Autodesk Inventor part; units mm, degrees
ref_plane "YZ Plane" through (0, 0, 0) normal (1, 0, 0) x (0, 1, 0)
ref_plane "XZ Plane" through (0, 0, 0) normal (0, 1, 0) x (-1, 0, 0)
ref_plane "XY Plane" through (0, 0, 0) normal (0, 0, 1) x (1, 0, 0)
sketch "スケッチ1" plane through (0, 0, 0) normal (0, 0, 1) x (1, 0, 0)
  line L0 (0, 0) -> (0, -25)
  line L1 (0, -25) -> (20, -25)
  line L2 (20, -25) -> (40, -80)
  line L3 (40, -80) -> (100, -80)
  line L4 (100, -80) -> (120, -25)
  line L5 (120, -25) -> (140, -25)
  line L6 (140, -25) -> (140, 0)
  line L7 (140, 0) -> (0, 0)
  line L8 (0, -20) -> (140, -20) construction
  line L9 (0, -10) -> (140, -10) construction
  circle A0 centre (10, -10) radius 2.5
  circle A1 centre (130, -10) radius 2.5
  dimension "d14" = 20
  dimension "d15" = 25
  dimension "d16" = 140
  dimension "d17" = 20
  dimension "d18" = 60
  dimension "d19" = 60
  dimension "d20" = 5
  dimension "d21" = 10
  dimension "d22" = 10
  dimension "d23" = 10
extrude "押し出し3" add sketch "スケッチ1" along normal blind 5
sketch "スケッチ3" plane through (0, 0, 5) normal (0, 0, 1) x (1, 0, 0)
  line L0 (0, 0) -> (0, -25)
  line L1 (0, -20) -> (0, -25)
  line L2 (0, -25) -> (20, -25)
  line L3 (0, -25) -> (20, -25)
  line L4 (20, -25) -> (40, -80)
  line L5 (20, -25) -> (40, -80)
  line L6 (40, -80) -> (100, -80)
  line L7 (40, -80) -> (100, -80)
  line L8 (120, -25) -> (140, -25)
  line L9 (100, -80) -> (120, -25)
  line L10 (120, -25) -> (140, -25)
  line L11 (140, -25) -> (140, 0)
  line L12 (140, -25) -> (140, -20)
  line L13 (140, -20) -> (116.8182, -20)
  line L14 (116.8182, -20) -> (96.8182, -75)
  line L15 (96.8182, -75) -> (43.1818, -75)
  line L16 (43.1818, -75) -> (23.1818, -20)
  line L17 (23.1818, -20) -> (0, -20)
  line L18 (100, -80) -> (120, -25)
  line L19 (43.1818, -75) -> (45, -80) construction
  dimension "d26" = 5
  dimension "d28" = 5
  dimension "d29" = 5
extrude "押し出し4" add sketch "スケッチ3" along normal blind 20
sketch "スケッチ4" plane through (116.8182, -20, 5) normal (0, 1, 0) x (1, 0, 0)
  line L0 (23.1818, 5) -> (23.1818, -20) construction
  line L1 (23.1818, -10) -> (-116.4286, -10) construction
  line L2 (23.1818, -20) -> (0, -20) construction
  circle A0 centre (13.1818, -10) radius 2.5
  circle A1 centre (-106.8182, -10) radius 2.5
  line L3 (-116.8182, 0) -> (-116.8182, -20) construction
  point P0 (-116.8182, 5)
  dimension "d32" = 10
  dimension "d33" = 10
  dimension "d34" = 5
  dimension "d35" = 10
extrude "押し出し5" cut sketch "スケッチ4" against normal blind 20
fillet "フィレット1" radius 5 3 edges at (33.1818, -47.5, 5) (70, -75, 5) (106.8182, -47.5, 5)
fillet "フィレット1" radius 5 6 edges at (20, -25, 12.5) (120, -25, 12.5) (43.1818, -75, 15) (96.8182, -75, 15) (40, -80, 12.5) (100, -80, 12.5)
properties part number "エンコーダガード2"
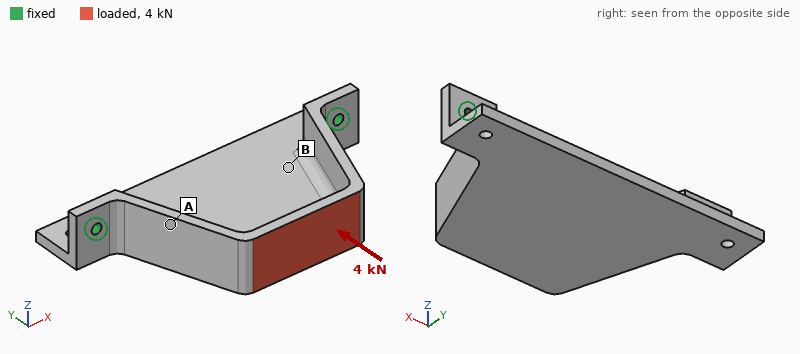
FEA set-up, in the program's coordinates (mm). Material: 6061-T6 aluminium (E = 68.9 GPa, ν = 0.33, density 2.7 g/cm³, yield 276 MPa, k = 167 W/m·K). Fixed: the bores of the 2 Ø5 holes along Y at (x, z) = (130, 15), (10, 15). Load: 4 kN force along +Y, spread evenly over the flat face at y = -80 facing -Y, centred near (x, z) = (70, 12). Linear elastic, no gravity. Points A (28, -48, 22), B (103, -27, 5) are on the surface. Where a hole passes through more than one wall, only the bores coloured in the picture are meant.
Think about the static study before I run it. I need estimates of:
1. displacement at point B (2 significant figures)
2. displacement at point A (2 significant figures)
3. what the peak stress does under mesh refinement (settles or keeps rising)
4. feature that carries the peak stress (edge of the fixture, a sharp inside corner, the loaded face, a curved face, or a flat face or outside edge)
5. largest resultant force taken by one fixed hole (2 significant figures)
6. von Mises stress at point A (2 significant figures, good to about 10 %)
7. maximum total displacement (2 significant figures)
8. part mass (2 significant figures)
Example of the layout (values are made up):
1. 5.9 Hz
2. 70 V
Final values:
1. 0.033 mm
2. 0.039 mm
3. keeps rising
4. edge of the fixture
5. 2.1 kN
6. 27 MPa
7. 0.14 mm
8. 160 g
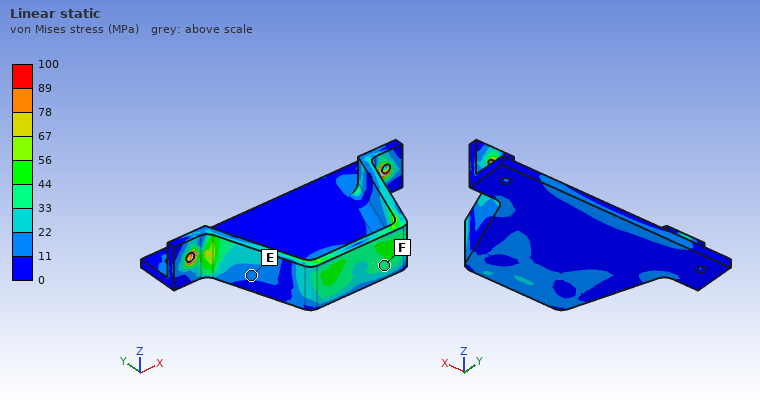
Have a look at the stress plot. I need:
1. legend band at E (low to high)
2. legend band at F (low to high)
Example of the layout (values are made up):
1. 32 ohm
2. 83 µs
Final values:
1. 11 to 22 MPa
2. 33 to 44 MPa
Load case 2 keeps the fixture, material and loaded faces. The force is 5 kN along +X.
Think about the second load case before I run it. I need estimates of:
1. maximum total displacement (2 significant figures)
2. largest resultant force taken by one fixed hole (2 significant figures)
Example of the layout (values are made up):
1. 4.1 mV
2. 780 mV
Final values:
1. 0.45 mm
2. 3.5 kN
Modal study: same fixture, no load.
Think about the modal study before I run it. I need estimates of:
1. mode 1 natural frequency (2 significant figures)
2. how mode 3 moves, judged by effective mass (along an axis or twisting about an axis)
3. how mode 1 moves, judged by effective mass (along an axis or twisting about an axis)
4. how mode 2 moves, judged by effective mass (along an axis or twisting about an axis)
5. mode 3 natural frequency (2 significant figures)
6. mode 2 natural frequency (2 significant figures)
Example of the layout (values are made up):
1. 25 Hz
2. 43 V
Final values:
1. 1000 Hz
2. along Z
3. along Z
4. along X
5. 2600 Hz
6. 2300 Hz
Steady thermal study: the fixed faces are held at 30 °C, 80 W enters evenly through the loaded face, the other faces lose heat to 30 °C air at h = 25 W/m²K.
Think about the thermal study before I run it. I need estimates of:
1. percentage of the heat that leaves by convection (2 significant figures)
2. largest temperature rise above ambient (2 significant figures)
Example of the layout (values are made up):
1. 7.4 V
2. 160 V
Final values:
1. 27 %
2. 76 K
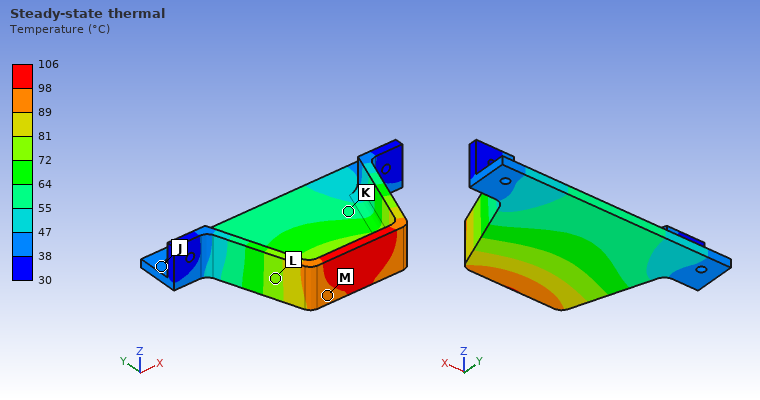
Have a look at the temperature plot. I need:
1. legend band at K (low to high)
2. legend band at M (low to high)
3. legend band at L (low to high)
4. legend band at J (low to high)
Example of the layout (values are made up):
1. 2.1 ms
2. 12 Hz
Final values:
1. 55 to 64 °C
2. 89 to 98 °C
3. 72 to 81 °C
4. 38 to 47 °C
